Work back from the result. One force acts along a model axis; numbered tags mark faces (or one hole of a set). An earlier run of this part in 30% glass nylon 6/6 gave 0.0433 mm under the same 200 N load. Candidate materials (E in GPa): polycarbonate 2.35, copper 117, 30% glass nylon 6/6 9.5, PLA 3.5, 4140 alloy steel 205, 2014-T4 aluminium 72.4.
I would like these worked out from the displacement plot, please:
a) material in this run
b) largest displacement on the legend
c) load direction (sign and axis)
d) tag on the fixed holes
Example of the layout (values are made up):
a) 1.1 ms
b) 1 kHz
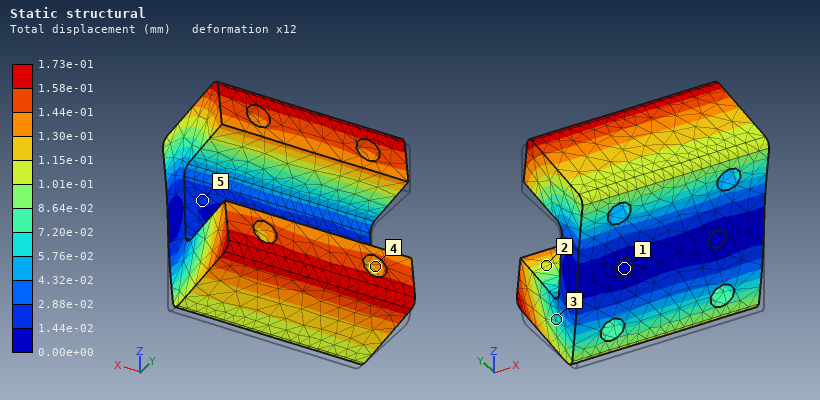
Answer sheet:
a) polycarbonate
b) 1.73e-01 mm
c) +Z
d) 1
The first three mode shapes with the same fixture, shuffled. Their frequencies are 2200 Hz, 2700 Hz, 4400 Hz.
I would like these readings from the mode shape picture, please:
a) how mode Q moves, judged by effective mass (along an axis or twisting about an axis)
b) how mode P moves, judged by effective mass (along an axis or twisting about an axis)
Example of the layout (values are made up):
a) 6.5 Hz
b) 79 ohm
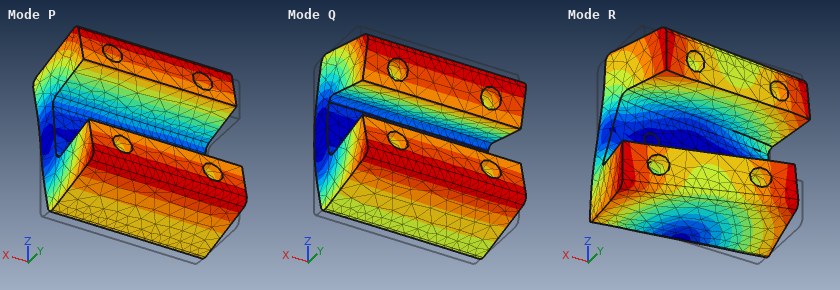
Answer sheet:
a) along Y
b) along Z
